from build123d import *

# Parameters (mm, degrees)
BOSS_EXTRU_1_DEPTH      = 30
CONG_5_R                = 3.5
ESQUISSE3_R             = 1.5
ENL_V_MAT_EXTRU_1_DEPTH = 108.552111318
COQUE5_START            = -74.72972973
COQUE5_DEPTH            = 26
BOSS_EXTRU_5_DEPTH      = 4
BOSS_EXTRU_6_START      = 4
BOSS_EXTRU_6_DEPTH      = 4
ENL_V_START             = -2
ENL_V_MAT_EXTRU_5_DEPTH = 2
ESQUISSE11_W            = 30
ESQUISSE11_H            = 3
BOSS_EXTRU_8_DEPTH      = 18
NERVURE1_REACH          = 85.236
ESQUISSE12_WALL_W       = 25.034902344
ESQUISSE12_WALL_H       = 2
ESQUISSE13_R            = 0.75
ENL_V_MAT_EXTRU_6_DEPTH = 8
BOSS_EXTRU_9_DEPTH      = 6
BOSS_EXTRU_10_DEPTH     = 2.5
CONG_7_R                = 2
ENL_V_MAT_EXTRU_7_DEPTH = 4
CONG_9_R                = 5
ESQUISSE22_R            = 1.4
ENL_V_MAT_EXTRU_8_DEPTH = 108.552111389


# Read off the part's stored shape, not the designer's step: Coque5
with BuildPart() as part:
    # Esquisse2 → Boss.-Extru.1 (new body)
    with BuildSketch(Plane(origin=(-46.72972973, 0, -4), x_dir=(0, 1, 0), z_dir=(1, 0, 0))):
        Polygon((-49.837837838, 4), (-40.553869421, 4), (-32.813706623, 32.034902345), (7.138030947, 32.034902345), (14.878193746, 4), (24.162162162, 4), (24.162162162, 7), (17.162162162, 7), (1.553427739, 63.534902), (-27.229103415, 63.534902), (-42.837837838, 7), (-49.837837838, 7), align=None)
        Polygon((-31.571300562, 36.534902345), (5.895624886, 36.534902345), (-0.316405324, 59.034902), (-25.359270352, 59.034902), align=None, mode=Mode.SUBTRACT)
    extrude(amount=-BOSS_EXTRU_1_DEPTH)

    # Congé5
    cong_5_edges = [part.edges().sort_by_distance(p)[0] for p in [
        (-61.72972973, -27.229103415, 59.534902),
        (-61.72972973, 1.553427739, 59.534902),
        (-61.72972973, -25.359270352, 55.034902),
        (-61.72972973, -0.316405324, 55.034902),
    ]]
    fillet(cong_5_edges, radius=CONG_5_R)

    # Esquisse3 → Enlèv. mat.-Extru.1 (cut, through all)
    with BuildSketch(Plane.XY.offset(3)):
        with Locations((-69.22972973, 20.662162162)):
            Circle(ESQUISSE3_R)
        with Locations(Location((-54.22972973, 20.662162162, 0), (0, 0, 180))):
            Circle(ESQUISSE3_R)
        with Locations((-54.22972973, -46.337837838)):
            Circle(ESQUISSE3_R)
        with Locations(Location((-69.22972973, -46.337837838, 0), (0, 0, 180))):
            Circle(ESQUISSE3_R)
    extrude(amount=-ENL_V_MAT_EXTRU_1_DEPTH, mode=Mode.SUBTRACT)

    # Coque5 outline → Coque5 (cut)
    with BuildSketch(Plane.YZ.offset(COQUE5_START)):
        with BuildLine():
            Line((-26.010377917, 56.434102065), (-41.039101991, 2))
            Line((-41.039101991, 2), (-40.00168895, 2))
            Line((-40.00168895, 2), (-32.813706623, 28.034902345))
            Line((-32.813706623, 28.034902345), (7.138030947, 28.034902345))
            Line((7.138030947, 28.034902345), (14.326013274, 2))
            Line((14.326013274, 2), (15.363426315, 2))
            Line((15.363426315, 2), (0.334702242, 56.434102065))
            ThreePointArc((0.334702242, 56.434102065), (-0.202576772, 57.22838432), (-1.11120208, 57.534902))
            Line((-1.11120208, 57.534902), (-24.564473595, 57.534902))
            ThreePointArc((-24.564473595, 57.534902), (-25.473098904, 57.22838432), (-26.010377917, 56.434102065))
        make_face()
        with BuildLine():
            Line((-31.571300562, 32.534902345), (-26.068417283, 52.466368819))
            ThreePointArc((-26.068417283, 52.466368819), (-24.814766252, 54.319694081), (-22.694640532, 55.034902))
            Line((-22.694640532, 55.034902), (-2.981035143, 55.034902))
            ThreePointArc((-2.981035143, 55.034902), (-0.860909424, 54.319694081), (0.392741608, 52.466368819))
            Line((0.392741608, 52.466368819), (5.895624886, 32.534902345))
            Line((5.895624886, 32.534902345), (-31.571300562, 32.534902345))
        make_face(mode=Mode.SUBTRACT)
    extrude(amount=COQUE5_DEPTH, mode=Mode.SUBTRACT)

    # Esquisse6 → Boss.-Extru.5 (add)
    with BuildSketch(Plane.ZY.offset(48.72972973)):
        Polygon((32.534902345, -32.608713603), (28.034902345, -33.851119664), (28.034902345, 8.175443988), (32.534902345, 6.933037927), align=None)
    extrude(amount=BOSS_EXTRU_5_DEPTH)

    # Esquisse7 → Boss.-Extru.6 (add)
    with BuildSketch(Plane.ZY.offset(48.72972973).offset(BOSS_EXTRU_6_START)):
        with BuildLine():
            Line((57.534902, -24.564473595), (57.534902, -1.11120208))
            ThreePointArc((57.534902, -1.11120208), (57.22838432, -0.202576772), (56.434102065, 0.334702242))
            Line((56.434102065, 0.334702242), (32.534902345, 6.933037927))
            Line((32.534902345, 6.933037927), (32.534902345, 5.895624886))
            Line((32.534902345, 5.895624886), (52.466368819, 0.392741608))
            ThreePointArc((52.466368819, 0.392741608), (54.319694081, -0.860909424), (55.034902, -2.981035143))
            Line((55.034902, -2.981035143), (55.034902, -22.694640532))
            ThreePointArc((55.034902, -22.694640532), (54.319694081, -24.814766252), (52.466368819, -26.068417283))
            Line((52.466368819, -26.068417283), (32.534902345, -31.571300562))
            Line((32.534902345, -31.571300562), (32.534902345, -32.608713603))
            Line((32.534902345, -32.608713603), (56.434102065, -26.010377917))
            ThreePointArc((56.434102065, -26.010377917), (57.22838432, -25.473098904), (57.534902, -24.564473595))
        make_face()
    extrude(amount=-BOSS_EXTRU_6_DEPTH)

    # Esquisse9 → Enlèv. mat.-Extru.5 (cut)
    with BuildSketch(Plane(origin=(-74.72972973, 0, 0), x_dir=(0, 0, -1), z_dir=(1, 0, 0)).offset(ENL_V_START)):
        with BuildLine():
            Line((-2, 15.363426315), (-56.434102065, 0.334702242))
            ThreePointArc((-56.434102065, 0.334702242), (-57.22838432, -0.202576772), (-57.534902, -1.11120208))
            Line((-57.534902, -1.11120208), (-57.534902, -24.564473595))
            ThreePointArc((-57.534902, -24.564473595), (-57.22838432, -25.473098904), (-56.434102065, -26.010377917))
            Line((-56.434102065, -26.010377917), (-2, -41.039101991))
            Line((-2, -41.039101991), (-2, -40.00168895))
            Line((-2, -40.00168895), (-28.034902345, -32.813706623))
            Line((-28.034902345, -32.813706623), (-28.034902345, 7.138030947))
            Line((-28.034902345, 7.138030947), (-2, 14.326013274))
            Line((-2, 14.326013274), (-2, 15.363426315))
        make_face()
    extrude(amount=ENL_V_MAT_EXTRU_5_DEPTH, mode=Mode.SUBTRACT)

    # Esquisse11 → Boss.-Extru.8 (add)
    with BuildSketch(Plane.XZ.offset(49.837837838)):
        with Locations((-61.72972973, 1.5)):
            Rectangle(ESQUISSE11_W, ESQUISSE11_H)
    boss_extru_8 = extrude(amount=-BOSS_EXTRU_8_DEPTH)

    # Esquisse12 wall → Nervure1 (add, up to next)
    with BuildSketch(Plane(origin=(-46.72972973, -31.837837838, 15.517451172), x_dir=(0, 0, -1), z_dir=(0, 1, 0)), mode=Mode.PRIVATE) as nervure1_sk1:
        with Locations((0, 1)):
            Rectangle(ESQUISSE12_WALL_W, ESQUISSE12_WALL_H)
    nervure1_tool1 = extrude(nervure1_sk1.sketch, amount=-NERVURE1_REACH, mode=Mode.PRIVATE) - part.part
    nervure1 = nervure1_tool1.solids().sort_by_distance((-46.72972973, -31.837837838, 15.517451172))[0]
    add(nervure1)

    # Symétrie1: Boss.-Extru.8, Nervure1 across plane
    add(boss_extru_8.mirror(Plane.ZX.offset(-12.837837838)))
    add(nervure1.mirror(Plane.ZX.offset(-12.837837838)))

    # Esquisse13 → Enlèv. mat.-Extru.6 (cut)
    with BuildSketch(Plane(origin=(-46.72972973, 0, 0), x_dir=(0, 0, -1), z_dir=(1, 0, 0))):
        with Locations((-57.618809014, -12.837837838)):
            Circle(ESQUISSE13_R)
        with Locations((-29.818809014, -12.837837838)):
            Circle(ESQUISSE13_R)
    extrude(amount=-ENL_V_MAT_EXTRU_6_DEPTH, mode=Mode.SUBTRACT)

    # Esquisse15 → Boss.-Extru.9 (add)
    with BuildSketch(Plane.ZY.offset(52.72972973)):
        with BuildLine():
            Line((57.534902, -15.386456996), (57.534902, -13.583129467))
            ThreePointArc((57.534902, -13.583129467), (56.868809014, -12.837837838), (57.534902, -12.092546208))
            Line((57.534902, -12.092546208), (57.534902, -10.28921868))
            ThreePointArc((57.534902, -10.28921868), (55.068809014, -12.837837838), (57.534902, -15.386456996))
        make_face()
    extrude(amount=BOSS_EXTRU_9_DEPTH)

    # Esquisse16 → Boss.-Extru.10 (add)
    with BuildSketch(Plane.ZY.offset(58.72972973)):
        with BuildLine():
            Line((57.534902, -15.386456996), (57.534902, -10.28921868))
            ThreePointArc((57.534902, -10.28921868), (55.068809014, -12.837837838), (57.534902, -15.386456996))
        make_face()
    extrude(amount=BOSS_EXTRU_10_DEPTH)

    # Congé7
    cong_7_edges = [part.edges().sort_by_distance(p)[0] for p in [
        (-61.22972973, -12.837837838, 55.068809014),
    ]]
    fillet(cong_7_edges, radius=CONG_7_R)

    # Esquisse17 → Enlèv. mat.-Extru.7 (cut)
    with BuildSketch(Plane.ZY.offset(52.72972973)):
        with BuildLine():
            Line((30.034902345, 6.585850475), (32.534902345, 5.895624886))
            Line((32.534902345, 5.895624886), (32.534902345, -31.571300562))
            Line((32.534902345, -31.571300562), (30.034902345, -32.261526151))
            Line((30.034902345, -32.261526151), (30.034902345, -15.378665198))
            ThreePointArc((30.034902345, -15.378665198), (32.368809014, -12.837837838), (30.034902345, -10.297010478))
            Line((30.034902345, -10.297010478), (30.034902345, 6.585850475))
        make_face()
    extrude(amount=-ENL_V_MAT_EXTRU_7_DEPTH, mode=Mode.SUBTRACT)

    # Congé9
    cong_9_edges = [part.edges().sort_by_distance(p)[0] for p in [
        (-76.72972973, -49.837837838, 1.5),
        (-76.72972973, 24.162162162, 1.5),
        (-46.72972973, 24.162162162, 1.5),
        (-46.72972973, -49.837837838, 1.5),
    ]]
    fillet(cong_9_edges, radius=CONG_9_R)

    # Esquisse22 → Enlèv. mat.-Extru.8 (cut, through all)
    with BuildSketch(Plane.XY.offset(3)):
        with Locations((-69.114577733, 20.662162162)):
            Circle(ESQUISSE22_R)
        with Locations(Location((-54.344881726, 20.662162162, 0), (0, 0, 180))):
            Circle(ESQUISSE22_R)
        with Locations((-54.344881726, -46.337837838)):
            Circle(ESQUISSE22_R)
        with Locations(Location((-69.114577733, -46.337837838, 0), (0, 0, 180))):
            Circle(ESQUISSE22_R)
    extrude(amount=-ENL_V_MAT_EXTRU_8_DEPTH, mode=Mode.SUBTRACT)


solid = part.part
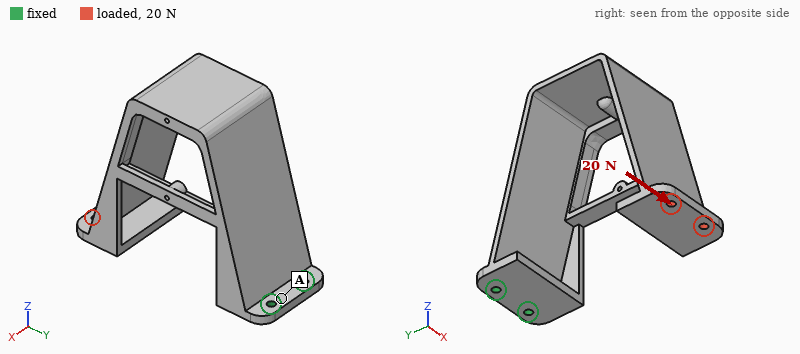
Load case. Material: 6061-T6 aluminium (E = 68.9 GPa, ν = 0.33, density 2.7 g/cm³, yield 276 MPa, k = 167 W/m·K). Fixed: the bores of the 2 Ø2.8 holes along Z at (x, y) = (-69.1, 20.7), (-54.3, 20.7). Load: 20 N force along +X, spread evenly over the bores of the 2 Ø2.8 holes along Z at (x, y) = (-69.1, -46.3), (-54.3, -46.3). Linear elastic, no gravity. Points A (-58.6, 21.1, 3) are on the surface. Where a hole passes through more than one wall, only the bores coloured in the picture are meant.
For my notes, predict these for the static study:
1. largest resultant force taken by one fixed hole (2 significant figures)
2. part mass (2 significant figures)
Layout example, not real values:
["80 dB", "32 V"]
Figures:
["82 N", "37 g"]
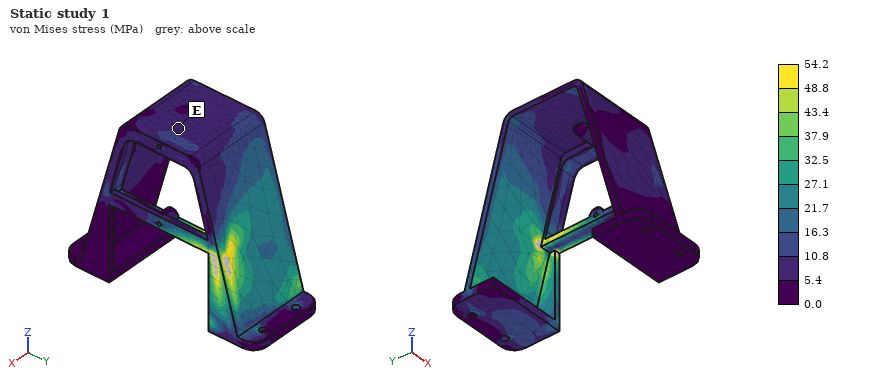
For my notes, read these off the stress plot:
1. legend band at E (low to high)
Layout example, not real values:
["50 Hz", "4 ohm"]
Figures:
["5.4 to 10.8 MPa"]
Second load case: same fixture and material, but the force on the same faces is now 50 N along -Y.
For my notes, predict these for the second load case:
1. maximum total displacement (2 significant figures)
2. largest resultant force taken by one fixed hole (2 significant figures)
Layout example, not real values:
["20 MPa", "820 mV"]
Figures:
["1.0 mm", "28 N"]
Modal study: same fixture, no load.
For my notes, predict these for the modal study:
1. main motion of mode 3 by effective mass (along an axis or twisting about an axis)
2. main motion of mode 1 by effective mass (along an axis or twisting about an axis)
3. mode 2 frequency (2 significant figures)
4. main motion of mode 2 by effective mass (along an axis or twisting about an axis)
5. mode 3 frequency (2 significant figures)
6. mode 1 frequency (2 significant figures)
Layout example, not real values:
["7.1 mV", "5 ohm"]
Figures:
["along Y", "along Z", "250 Hz", "along X", "680 Hz", "210 Hz"]
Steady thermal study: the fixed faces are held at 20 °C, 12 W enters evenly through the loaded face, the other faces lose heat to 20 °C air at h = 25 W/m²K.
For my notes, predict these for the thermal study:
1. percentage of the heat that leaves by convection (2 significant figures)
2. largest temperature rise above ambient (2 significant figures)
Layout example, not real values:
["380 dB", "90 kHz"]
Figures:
["70 %", "66 K"]
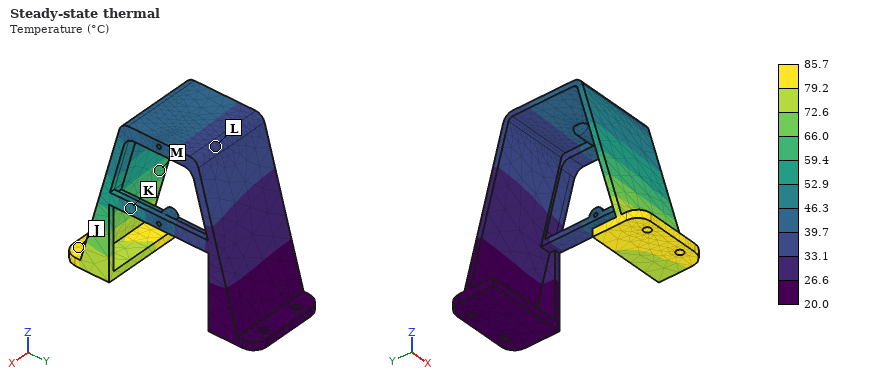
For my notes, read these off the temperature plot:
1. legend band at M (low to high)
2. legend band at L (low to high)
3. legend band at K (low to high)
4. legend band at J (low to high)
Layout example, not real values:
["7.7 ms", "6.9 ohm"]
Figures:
["59.4 to 66.0 °C", "33.1 to 39.7 °C", "46.3 to 52.9 °C", "79.2 to 85.7 °C"]
